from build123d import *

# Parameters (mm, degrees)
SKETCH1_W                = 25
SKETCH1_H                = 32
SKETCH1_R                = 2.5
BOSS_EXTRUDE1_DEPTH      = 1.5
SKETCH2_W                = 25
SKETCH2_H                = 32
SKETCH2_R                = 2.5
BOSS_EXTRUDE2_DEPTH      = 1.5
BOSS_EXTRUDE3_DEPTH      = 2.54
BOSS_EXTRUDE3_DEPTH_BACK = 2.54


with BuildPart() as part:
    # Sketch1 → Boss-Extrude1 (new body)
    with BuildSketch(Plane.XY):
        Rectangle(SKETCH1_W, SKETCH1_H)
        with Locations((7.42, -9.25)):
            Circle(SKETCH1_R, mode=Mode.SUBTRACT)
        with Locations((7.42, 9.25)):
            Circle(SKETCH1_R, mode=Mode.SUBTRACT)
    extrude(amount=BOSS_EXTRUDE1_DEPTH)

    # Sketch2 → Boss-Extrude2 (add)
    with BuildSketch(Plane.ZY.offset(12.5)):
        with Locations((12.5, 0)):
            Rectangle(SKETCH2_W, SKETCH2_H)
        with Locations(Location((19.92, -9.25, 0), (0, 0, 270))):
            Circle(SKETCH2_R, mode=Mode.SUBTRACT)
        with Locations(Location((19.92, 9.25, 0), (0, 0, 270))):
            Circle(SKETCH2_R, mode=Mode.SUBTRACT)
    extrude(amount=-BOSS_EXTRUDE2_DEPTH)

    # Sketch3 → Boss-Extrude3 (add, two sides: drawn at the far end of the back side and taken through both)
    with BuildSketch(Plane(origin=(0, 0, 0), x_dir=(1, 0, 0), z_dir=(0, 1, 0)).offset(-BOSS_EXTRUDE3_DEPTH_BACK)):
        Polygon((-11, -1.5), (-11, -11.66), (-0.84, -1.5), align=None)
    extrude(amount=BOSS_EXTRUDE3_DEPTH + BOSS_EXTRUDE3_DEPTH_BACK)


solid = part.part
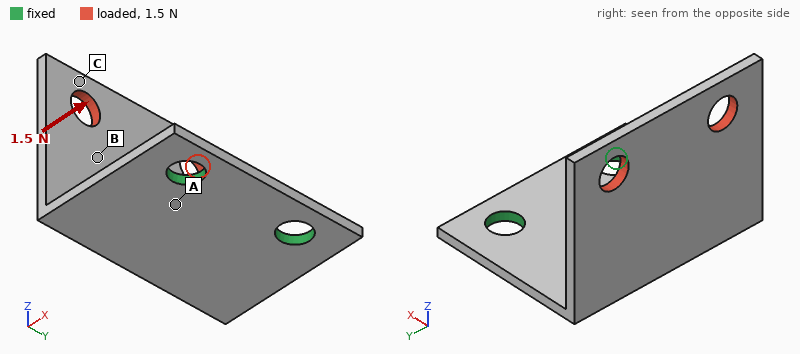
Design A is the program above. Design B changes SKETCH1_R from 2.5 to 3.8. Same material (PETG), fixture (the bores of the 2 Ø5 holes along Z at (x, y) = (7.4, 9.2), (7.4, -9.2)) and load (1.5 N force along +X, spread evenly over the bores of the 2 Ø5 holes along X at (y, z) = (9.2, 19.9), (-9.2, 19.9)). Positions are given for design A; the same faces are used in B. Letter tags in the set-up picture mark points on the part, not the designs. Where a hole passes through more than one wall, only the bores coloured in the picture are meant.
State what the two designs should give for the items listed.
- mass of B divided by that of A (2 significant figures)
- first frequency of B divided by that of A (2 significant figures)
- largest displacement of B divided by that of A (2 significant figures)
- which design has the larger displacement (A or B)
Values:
0.97
1.1
0.86
A
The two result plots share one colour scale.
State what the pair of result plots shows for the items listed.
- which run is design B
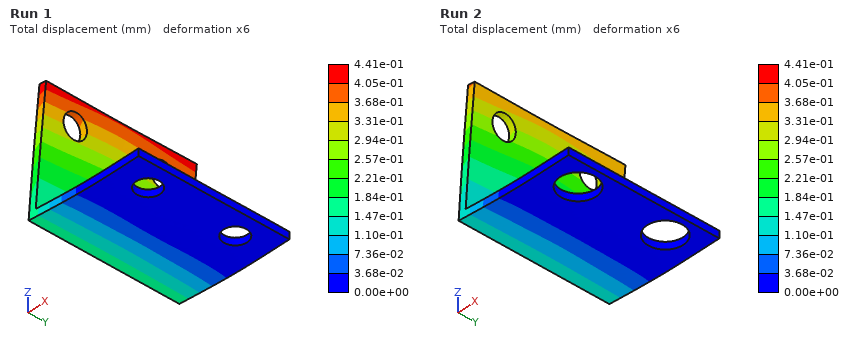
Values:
Run 2
